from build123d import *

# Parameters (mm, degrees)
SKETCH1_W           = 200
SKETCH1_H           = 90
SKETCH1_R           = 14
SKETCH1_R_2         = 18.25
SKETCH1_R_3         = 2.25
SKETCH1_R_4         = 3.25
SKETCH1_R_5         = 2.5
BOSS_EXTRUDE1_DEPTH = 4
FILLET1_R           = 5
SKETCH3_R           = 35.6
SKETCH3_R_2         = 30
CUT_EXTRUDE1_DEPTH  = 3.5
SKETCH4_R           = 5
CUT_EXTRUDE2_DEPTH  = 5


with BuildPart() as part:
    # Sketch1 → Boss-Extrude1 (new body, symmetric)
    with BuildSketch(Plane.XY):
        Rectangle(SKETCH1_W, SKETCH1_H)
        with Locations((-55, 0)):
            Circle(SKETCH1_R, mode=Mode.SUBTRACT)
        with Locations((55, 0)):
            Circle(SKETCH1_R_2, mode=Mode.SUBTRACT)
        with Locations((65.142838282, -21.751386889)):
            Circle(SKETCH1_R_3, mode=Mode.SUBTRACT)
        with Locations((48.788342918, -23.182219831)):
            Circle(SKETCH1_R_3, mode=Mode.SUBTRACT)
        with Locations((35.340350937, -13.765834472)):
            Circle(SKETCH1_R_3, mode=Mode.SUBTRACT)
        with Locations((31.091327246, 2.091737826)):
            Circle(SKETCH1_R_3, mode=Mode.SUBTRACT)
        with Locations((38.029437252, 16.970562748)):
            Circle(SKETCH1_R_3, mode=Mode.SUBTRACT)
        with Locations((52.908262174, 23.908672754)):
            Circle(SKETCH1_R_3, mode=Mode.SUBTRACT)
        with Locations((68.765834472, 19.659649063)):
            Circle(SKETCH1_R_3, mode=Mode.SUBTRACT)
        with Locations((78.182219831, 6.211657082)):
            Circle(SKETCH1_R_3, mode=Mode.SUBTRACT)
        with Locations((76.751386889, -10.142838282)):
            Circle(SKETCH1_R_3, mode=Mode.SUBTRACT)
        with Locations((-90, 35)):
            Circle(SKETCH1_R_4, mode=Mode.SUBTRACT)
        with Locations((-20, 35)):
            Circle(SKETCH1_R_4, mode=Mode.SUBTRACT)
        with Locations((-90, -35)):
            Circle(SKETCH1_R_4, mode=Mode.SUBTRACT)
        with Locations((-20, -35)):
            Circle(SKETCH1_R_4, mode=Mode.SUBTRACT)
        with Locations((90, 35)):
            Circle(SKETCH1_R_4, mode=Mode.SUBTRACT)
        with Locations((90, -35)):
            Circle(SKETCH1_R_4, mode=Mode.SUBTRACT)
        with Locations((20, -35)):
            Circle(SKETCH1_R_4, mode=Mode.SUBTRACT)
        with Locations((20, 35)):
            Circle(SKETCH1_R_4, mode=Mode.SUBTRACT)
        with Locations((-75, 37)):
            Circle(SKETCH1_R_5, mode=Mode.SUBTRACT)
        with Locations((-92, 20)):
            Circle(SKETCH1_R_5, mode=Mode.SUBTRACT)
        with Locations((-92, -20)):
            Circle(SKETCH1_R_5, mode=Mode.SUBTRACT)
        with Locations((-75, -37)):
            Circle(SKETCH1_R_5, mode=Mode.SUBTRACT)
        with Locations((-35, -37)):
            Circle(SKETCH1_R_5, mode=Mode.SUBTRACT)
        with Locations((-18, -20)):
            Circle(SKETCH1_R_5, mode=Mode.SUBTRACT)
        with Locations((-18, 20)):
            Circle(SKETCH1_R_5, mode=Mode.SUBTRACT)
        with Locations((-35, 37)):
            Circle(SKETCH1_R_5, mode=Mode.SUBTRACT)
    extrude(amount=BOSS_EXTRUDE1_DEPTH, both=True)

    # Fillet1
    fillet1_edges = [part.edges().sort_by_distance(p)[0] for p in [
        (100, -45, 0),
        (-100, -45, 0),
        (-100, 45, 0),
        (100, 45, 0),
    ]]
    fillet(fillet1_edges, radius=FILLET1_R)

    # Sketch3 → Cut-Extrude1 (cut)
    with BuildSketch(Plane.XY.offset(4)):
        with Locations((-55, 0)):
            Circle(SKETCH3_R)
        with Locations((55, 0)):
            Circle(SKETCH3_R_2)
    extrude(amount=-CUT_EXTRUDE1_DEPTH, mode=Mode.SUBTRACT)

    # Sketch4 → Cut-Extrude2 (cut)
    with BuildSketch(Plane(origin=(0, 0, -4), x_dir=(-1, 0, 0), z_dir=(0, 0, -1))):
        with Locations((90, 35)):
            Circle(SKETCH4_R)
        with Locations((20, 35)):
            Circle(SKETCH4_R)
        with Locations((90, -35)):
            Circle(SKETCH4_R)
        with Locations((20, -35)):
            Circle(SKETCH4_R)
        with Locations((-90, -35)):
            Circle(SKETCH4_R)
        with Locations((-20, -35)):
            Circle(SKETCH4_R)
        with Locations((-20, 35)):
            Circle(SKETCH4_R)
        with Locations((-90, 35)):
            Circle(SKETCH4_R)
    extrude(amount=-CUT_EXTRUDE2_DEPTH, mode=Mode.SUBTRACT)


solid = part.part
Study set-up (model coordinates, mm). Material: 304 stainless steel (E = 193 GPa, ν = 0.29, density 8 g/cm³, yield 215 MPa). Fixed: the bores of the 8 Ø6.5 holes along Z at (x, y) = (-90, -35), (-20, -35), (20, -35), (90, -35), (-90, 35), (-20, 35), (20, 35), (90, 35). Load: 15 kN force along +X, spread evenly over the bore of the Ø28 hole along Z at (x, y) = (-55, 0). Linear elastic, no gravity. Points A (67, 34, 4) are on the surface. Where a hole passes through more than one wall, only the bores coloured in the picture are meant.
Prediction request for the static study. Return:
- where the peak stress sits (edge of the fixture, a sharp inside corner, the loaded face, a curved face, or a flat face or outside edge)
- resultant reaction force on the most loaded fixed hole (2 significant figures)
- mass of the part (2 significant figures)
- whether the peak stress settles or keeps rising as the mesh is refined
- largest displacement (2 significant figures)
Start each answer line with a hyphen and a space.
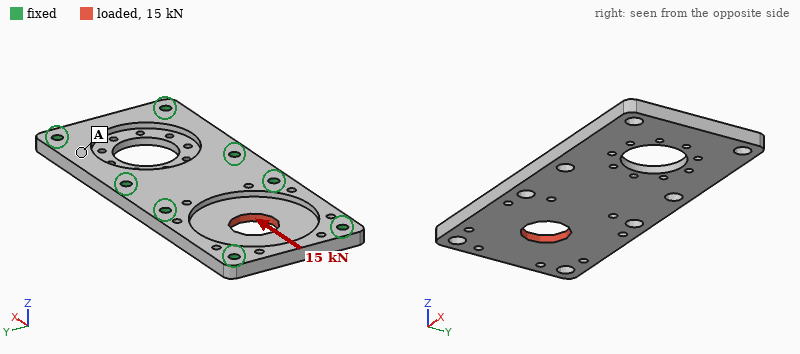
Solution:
- edge of the fixture
- 3.0 kN
- 850 g
- keeps rising
- 15 µm
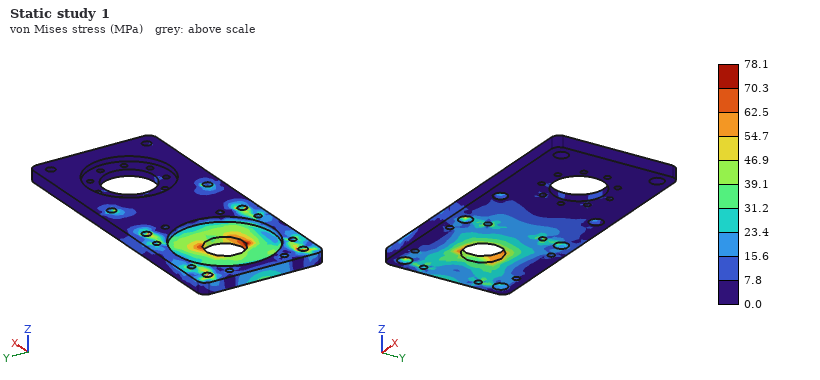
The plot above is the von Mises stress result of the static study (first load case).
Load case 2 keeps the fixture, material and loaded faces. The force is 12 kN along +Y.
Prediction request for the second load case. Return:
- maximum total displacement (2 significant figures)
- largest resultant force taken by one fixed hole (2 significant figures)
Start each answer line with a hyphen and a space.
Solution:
- 12 µm
- 3.0 kN
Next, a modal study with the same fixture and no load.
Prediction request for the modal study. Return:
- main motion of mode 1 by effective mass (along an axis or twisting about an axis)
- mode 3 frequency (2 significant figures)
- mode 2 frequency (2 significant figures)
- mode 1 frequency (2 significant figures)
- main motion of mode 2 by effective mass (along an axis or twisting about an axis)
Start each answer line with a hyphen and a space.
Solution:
- along Z
- 6100 Hz
- 5500 Hz
- 5000 Hz
- along Z
